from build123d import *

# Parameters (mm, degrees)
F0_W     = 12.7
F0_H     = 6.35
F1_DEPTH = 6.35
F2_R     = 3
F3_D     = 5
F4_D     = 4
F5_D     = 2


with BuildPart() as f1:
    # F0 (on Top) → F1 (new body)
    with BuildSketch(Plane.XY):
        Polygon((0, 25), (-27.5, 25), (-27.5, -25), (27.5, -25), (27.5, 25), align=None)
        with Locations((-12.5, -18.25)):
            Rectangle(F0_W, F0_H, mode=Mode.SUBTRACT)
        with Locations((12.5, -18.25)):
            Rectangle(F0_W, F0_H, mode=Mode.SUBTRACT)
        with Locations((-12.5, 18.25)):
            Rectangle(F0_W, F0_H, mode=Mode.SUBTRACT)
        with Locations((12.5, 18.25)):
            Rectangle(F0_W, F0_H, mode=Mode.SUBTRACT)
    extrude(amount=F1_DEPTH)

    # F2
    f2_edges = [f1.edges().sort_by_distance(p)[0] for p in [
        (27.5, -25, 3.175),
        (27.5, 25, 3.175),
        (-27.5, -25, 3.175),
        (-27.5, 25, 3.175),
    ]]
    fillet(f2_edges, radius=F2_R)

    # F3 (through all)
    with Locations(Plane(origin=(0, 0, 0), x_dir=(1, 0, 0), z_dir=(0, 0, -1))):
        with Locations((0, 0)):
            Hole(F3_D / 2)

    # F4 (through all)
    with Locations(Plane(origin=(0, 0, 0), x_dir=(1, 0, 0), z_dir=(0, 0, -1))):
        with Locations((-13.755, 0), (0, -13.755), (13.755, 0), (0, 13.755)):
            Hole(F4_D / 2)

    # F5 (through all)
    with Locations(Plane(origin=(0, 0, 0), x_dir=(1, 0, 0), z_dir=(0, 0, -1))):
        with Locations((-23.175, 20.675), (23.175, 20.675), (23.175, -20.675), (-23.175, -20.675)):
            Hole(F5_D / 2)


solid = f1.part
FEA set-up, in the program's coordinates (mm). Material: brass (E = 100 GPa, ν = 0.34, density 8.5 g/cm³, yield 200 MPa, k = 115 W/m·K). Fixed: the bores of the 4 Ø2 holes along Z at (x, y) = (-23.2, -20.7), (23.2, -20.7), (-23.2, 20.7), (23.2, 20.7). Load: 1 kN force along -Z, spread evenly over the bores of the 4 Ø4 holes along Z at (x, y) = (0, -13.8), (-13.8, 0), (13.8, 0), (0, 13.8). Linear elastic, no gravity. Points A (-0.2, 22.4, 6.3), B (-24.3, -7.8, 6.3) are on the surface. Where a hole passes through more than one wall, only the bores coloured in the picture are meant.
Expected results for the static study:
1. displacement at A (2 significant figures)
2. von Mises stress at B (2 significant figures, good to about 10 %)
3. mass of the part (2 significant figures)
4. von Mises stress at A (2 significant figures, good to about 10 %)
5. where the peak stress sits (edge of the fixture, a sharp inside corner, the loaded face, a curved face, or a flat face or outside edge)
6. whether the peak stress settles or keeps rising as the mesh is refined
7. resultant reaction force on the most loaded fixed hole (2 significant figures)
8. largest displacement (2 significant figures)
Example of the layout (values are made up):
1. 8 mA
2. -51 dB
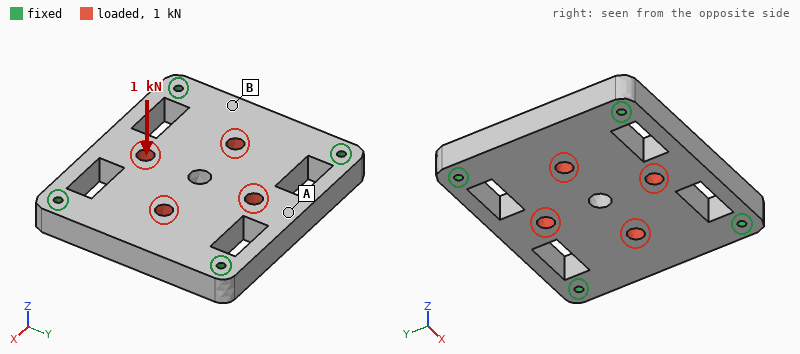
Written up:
1. 8.6 µm
2. 6.4 MPa
3. 130 g
4. 14 MPa
5. edge of the fixture
6. keeps rising
7. 250 N
8. 14 µm
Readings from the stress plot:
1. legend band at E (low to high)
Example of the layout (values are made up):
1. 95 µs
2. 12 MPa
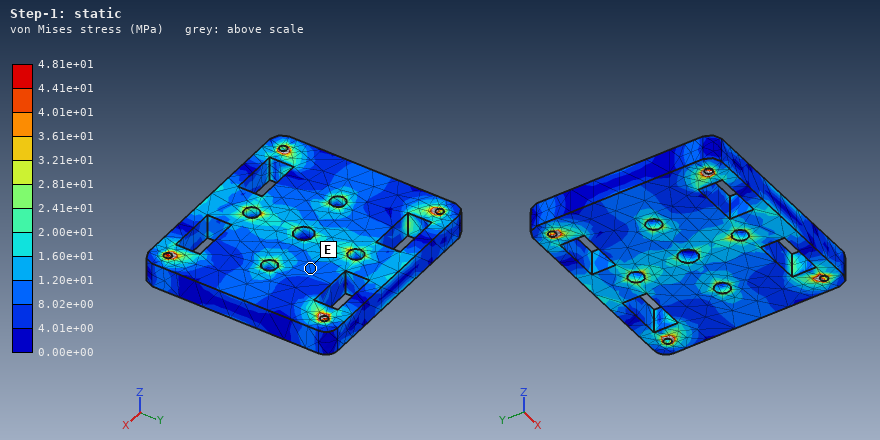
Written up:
1. 8.02e+00 to 1.20e+01 MPa
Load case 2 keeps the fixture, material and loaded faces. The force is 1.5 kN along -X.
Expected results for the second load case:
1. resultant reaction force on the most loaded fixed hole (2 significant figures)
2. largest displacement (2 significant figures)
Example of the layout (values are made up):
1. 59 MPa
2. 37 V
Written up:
1. 400 N
2. 2.9 µm
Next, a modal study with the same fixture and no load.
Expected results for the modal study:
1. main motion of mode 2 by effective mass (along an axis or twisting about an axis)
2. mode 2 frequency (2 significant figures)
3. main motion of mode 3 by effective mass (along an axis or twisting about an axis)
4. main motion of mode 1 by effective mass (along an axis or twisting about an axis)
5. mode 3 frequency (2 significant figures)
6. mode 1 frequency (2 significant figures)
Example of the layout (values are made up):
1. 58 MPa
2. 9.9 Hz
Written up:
1. twisting about X
2. 8900 Hz
3. twisting about Y
4. along Z
5. 10 kHz
6. 5700 Hz
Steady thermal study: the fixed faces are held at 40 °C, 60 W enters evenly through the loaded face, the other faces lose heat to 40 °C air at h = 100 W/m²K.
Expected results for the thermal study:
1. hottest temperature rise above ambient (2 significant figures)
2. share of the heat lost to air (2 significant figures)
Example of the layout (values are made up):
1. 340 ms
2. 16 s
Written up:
1. 29 K
2. 19 %
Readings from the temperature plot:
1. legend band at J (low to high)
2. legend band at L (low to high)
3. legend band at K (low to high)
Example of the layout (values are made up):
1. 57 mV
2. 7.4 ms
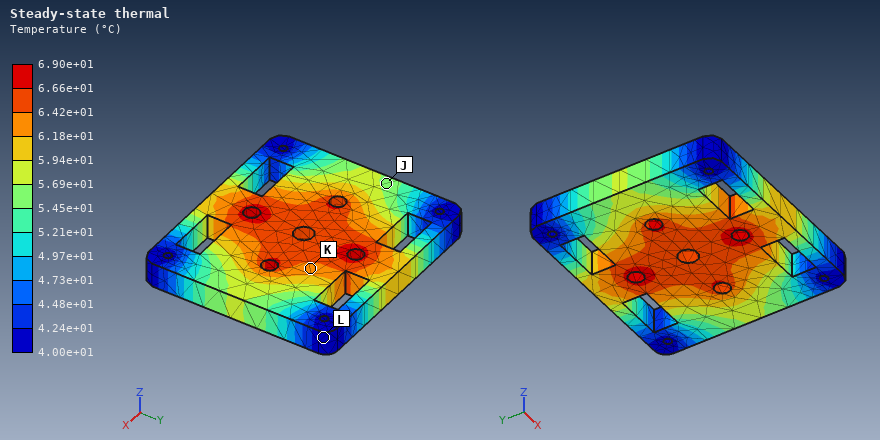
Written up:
1. 5.45e+01 to 5.69e+01 °C
2. 4.00e+01 to 4.24e+01 °C
3. 6.18e+01 to 6.42e+01 °C
